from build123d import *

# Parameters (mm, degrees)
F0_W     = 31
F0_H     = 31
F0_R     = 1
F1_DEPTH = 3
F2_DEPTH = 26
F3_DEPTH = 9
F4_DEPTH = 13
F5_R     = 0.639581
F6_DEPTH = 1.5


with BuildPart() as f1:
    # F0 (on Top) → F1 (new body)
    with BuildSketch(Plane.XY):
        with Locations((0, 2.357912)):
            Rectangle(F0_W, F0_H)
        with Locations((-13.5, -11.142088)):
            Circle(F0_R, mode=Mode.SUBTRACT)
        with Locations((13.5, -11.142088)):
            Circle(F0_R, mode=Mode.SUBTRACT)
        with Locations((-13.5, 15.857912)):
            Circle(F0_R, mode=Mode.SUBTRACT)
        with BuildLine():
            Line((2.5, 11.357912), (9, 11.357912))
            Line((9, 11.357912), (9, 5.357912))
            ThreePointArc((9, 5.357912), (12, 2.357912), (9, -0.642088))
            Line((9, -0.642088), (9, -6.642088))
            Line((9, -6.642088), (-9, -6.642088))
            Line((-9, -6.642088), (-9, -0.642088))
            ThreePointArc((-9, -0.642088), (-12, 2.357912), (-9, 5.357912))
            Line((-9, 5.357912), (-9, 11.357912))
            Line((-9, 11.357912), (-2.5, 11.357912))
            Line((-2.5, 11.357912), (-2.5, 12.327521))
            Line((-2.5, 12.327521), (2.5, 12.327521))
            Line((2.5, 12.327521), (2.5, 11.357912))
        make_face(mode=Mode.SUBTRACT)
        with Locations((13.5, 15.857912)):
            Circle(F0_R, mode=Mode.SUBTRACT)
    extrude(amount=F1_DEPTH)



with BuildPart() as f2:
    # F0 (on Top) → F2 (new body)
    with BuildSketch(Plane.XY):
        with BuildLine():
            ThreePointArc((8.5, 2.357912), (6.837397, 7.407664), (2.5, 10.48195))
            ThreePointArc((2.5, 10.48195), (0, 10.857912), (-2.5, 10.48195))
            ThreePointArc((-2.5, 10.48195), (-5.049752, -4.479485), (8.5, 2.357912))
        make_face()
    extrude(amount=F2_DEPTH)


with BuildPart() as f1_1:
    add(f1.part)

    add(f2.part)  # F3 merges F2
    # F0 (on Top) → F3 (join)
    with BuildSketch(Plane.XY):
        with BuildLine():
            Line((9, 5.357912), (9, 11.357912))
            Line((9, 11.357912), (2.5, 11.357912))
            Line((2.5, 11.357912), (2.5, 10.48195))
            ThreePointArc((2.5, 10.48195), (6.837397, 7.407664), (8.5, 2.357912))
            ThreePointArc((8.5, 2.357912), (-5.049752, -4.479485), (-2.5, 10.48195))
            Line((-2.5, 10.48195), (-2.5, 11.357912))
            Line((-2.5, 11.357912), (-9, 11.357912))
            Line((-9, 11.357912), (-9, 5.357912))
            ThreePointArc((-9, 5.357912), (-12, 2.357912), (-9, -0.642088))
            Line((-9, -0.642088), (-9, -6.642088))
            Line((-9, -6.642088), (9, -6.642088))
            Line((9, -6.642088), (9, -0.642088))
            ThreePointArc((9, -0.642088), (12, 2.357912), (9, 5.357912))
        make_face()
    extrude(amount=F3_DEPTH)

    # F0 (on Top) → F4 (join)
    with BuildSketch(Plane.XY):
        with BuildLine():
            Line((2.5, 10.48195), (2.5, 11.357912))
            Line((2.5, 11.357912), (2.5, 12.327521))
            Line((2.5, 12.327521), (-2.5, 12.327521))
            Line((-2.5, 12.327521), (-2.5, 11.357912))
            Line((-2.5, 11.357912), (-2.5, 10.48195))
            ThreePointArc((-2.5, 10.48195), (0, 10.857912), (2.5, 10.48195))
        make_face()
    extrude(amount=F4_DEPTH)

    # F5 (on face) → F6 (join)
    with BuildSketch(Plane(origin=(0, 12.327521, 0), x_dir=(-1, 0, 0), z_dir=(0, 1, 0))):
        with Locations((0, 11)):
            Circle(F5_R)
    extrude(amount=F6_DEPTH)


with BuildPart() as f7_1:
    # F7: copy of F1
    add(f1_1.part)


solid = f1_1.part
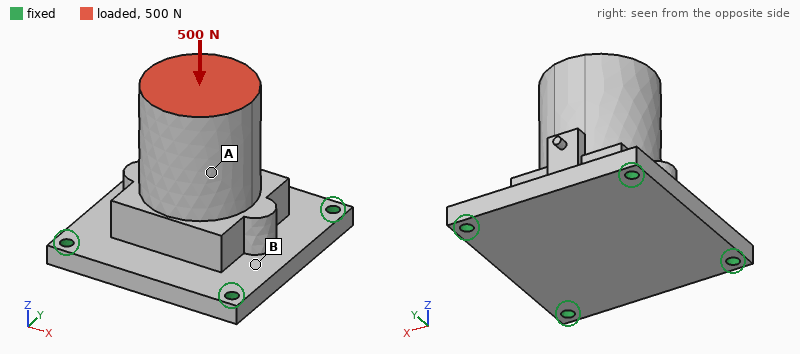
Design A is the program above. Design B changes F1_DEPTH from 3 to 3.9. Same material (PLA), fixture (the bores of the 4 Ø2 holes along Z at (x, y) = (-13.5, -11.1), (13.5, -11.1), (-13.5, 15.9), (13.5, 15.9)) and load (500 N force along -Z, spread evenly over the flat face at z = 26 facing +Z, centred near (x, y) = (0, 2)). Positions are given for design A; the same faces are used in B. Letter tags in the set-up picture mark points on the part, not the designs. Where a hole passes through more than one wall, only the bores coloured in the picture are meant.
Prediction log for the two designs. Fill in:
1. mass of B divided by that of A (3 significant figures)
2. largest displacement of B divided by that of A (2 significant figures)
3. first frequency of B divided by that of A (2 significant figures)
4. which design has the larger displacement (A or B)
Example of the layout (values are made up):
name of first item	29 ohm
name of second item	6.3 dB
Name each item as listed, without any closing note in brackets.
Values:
mass of B divided by that of A	1.06
largest displacement of B divided by that of A	0.64
first frequency of B divided by that of A	1.3
which design has the larger displacement	A
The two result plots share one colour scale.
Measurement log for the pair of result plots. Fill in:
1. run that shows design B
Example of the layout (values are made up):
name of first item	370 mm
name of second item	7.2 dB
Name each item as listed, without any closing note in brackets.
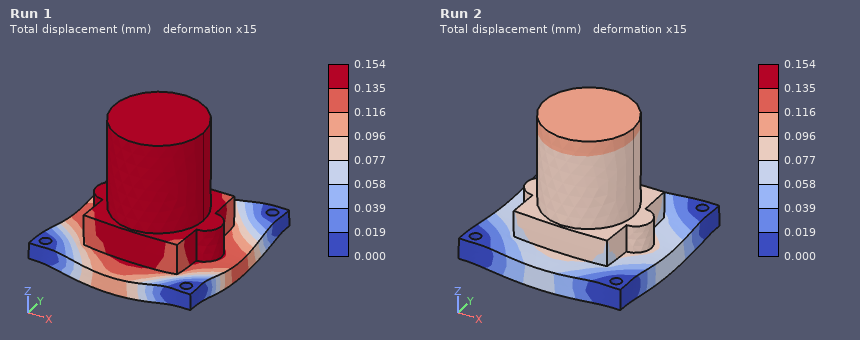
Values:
run that shows design B	Run 2
